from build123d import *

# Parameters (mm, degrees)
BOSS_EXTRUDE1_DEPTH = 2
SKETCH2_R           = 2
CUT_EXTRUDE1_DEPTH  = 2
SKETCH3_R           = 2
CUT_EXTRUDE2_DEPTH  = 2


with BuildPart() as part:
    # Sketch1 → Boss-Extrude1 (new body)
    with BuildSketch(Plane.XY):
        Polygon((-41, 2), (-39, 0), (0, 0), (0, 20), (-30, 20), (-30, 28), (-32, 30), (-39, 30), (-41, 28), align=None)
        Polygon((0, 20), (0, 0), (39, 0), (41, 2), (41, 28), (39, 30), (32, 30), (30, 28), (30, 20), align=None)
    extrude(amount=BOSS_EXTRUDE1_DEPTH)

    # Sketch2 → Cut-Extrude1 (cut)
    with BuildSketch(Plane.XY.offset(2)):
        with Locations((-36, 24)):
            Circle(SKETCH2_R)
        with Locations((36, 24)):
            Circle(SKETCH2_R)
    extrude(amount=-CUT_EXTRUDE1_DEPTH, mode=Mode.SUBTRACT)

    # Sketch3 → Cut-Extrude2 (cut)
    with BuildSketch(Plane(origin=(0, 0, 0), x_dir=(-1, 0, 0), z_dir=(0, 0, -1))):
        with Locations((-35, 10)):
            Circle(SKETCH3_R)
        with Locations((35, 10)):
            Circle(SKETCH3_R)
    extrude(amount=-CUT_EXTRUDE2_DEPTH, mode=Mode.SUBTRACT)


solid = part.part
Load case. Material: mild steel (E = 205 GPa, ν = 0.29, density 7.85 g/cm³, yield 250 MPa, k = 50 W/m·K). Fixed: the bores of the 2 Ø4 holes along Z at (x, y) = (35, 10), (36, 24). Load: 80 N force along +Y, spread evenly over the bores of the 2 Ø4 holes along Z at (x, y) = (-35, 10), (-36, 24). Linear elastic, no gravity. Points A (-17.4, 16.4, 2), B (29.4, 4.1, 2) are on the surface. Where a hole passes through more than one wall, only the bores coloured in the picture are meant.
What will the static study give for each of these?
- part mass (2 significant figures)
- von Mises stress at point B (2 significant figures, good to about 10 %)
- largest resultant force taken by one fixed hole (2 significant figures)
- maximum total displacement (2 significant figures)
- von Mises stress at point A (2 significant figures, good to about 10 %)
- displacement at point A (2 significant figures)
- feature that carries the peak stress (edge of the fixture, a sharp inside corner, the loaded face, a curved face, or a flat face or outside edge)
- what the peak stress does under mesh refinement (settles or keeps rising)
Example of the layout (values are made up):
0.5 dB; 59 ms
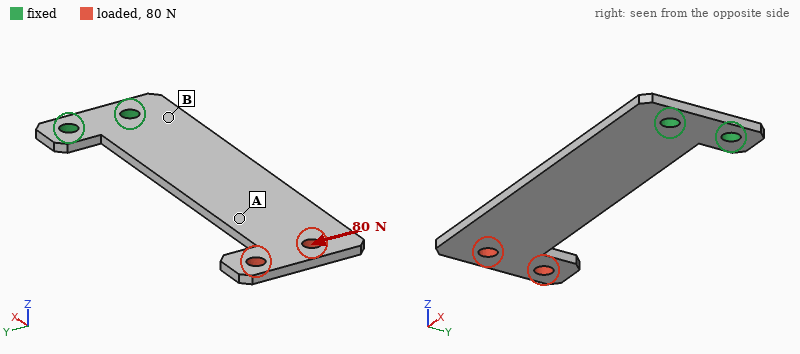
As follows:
28 g; 23 MPa; 340 N; 53 µm; 7.6 MPa; 30 µm; a sharp inside corner; keeps rising
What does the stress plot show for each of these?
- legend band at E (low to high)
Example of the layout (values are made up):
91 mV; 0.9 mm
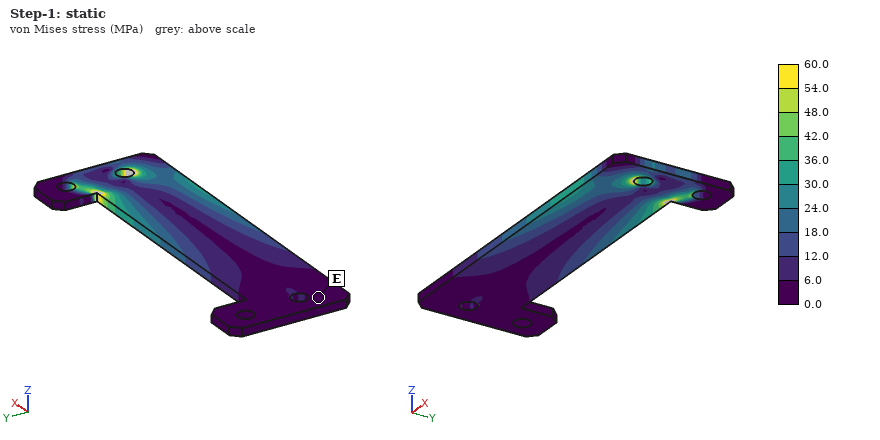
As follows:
0.0 to 6.0 MPa
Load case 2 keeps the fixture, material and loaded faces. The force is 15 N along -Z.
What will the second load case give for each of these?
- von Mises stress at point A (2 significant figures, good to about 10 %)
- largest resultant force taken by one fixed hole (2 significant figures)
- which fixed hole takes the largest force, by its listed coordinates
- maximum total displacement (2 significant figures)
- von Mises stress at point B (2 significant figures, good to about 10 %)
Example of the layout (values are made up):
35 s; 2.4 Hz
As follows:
23 MPa; 23 N; (35, 10); 0.71 mm; 64 MPa
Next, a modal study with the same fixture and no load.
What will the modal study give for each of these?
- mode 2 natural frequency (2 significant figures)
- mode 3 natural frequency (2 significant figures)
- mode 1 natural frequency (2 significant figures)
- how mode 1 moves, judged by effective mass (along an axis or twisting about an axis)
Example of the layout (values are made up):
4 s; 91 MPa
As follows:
1500 Hz; 1900 Hz; 270 Hz; along Z
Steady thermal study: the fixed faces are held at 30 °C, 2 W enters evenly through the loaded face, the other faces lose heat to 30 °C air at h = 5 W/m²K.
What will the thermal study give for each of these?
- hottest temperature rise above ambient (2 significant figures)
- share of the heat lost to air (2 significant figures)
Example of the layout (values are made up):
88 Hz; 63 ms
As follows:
64 K; 28 %
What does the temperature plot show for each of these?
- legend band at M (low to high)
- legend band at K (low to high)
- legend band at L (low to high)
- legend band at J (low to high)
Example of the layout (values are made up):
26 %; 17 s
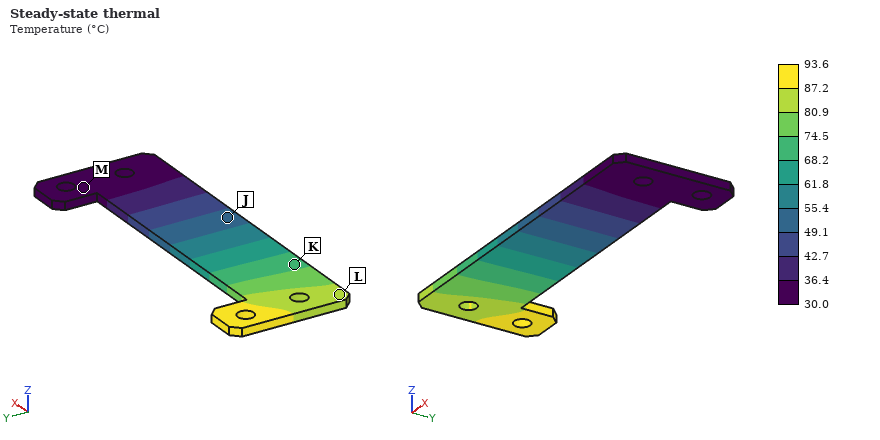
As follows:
30.0 to 36.4 °C; 68.2 to 74.5 °C; 80.9 to 87.2 °C; 49.1 to 55.4 °C
